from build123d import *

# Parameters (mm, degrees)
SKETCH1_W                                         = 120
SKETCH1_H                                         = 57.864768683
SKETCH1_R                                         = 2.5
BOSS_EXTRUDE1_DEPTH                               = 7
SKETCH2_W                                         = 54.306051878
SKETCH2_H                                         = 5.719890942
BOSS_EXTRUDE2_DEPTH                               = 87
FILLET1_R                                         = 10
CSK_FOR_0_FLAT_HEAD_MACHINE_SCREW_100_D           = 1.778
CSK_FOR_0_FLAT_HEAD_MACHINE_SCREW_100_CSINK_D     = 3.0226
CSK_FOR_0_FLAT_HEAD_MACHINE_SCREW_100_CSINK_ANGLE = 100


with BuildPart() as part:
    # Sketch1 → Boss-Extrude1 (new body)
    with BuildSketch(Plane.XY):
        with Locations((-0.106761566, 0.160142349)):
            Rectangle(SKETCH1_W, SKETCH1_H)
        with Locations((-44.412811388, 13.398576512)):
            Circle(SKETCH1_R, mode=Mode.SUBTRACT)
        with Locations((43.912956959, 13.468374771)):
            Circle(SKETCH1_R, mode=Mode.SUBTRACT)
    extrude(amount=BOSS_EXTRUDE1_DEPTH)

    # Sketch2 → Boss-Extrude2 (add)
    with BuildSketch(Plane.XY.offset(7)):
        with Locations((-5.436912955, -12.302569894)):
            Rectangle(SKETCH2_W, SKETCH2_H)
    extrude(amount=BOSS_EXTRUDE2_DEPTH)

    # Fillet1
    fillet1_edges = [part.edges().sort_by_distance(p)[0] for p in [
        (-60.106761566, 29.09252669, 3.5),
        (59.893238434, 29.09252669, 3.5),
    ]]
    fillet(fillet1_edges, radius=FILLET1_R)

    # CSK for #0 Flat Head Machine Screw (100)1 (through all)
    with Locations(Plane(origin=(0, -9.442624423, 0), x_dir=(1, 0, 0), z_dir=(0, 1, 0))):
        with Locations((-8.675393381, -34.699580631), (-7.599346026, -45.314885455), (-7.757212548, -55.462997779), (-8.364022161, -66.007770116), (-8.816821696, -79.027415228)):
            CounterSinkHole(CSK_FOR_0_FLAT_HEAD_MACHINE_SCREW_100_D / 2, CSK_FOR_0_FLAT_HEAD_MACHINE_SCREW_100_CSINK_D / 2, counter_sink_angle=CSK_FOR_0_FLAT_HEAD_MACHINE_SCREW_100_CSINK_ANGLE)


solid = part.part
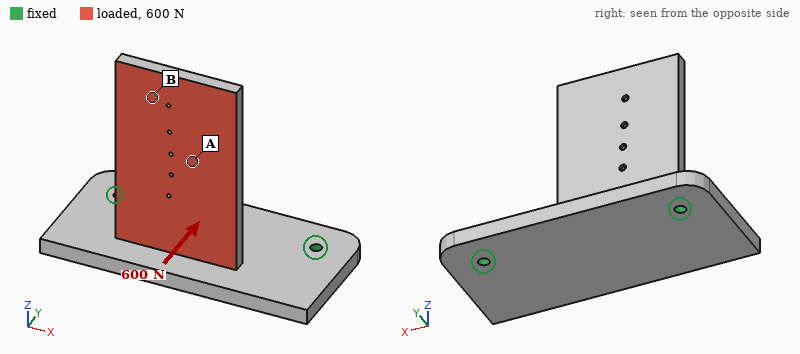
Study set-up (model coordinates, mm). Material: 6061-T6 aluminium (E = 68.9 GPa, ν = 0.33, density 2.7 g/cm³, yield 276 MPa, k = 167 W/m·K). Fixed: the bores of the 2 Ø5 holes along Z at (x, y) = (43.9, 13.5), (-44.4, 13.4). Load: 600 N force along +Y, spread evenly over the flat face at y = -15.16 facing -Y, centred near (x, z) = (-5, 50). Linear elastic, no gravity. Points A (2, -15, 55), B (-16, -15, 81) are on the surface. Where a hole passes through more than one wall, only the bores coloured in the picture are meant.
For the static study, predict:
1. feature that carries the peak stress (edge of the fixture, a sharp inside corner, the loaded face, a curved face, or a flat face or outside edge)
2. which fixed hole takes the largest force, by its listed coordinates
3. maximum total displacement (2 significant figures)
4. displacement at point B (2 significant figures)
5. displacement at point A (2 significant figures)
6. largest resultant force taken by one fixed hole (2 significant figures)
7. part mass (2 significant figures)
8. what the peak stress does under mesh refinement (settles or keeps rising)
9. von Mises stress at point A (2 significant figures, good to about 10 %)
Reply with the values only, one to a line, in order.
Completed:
edge of the fixture
(-44.4, 13.4)
1.3 mm
1.1 mm
0.62 mm
370 N
200 g
keeps rising
18 MPa
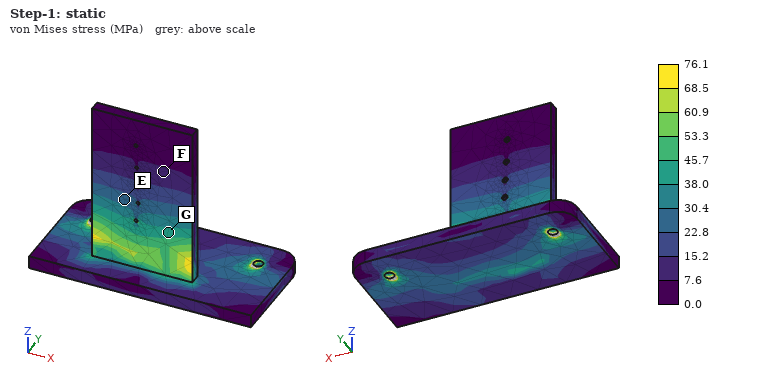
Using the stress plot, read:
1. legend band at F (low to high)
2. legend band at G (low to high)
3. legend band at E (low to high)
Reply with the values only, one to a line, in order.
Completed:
7.6 to 15.2 MPa
38.0 to 45.7 MPa
22.8 to 30.4 MPa
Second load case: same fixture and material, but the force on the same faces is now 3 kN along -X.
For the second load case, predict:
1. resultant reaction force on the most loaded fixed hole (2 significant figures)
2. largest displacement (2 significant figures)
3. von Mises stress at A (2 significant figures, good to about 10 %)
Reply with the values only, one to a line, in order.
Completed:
2.5 kN
0.48 mm
22 MPa
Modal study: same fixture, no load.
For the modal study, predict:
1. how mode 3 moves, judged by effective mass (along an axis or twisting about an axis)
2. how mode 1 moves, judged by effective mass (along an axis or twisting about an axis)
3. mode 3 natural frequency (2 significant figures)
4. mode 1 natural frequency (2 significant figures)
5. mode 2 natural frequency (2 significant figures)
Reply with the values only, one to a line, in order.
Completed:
along Z
along Y
1800 Hz
490 Hz
1600 Hz
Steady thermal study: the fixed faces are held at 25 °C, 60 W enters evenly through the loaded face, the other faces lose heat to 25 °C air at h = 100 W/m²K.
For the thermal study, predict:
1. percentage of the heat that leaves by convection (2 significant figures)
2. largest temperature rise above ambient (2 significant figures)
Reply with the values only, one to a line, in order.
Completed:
53 %
43 K
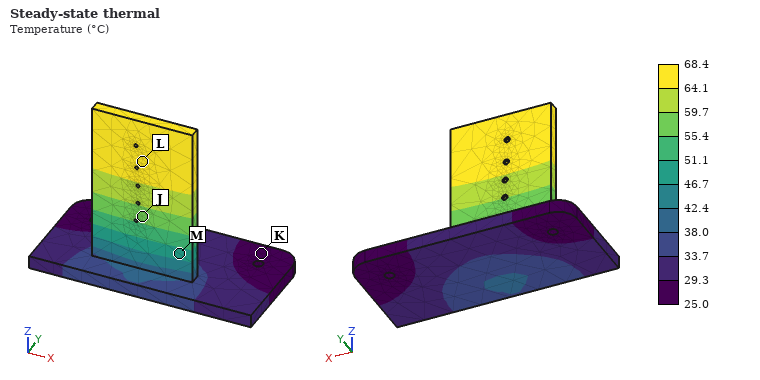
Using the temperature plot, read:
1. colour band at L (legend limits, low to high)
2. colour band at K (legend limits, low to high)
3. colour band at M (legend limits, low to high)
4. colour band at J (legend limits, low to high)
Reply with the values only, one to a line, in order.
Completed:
64.1 to 68.4 °C
25.0 to 29.3 °C
46.7 to 51.1 °C
55.4 to 59.7 °C
